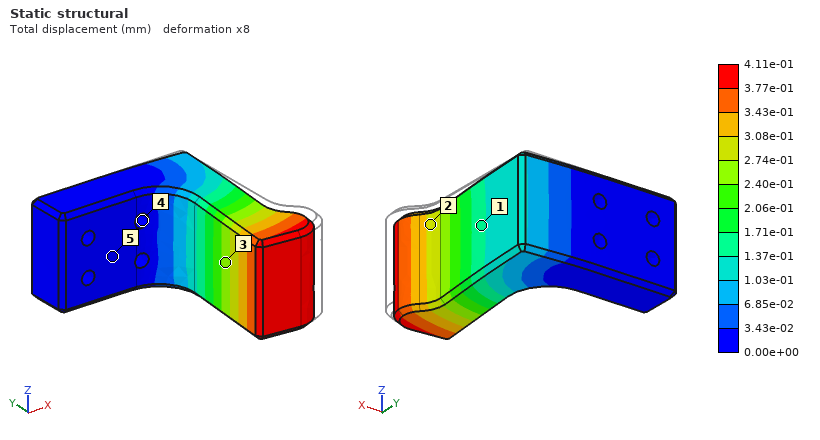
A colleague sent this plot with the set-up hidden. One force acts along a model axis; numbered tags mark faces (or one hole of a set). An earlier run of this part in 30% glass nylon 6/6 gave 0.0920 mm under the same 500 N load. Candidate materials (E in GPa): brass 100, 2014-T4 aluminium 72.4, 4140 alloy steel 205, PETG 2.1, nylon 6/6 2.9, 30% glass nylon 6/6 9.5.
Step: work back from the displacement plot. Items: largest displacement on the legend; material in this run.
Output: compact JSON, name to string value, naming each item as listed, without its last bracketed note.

{"largest displacement on the legend": "4.11e-01 mm", "material in this run": "PETG"}
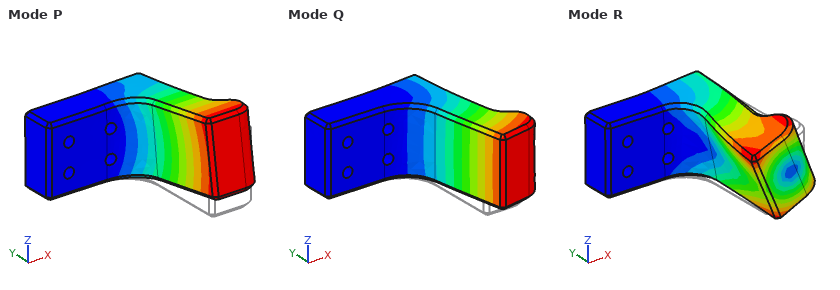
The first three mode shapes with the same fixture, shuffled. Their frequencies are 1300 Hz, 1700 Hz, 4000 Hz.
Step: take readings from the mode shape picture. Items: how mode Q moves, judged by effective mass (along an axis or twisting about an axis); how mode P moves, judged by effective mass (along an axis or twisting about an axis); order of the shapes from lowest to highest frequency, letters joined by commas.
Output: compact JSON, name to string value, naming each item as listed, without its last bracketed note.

{"how mode Q moves, judged by effective mass": "along X", "how mode P moves, judged by effective mass": "along Z", "order of the shapes from lowest to highest frequency, letters joined by commas": "Q, P, R"}
